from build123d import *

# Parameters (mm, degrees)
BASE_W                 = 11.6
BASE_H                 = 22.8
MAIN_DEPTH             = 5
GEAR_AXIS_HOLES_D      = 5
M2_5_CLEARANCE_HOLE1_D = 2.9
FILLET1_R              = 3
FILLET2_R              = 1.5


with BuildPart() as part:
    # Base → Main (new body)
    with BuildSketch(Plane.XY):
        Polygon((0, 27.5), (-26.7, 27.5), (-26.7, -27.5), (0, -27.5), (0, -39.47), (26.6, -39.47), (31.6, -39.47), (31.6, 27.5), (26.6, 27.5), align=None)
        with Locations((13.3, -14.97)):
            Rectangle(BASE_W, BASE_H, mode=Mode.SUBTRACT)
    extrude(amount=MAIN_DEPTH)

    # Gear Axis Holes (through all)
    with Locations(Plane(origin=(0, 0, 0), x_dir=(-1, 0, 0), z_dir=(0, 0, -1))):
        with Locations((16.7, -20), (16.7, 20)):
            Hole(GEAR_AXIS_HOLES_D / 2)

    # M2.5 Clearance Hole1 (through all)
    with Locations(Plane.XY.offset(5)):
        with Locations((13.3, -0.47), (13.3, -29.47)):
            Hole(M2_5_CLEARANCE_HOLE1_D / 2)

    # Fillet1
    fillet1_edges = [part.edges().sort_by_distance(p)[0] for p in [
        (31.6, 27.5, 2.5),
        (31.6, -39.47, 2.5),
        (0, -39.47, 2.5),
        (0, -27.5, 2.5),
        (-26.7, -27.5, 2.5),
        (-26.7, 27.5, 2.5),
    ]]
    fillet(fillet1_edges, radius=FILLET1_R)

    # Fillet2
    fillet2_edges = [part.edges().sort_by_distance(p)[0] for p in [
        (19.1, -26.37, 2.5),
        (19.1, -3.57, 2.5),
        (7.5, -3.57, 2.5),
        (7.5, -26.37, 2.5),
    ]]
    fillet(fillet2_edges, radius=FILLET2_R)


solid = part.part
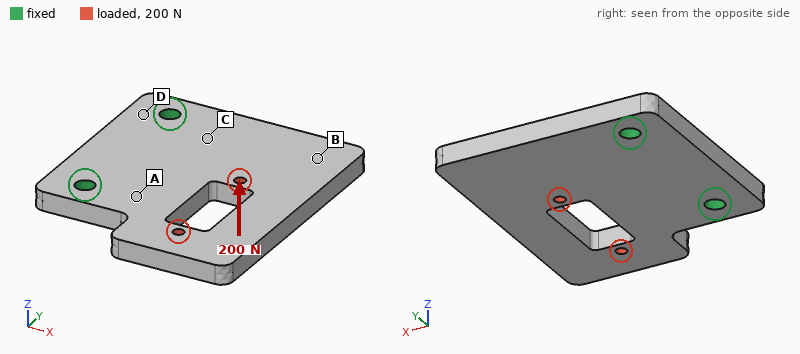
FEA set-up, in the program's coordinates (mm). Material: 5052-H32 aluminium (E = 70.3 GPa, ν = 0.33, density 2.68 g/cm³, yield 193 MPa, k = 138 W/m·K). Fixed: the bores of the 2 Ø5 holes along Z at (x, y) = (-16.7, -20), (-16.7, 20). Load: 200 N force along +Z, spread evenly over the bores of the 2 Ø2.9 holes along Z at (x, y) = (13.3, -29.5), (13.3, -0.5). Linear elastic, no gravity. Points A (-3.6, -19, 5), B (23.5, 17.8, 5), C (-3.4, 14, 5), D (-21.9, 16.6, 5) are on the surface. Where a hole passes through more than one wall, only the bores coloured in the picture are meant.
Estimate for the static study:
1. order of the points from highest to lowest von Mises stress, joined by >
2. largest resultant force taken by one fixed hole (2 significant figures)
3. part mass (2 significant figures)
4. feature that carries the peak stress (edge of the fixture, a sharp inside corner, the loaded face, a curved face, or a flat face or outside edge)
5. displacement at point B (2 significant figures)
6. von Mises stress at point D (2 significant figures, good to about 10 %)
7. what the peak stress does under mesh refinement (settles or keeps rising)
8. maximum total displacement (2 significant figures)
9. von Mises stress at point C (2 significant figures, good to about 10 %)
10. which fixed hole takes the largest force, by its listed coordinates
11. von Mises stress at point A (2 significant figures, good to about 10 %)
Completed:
A > C > D > B
170 N
44 g
edge of the fixture
0.061 mm
7.7 MPa
keeps rising
0.14 mm
12 MPa
(-16.7, -20)
19 MPa
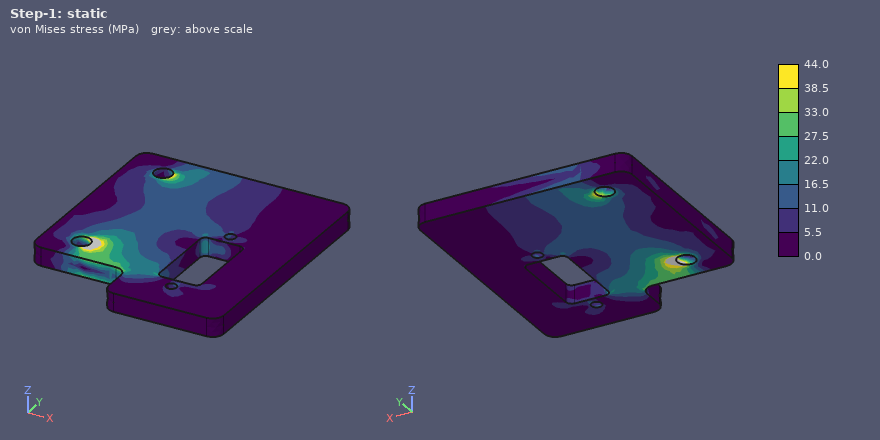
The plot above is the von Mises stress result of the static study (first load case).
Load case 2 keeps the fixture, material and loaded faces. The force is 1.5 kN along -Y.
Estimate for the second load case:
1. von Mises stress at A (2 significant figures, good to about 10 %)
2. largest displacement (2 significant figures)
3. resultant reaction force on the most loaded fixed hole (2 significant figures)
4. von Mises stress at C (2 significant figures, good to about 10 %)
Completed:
11 MPa
23 µm
1.3 kN
11 MPa
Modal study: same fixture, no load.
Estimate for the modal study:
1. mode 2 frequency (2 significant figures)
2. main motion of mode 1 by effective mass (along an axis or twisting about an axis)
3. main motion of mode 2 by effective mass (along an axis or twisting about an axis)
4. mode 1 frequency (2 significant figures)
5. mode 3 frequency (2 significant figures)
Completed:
2800 Hz
along Z
twisting about X
1500 Hz
6700 Hz
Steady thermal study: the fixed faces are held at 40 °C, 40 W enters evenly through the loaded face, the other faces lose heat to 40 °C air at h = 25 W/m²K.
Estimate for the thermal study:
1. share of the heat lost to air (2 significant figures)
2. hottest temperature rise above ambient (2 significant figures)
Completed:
12 %
59 K
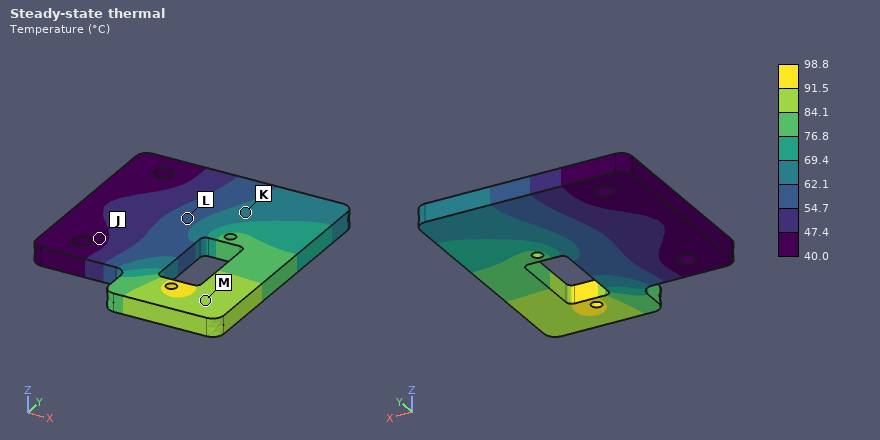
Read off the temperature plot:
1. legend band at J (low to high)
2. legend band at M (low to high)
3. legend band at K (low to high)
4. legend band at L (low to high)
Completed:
40.0 to 47.4 °C
84.1 to 91.5 °C
62.1 to 69.4 °C
54.7 to 62.1 °C
